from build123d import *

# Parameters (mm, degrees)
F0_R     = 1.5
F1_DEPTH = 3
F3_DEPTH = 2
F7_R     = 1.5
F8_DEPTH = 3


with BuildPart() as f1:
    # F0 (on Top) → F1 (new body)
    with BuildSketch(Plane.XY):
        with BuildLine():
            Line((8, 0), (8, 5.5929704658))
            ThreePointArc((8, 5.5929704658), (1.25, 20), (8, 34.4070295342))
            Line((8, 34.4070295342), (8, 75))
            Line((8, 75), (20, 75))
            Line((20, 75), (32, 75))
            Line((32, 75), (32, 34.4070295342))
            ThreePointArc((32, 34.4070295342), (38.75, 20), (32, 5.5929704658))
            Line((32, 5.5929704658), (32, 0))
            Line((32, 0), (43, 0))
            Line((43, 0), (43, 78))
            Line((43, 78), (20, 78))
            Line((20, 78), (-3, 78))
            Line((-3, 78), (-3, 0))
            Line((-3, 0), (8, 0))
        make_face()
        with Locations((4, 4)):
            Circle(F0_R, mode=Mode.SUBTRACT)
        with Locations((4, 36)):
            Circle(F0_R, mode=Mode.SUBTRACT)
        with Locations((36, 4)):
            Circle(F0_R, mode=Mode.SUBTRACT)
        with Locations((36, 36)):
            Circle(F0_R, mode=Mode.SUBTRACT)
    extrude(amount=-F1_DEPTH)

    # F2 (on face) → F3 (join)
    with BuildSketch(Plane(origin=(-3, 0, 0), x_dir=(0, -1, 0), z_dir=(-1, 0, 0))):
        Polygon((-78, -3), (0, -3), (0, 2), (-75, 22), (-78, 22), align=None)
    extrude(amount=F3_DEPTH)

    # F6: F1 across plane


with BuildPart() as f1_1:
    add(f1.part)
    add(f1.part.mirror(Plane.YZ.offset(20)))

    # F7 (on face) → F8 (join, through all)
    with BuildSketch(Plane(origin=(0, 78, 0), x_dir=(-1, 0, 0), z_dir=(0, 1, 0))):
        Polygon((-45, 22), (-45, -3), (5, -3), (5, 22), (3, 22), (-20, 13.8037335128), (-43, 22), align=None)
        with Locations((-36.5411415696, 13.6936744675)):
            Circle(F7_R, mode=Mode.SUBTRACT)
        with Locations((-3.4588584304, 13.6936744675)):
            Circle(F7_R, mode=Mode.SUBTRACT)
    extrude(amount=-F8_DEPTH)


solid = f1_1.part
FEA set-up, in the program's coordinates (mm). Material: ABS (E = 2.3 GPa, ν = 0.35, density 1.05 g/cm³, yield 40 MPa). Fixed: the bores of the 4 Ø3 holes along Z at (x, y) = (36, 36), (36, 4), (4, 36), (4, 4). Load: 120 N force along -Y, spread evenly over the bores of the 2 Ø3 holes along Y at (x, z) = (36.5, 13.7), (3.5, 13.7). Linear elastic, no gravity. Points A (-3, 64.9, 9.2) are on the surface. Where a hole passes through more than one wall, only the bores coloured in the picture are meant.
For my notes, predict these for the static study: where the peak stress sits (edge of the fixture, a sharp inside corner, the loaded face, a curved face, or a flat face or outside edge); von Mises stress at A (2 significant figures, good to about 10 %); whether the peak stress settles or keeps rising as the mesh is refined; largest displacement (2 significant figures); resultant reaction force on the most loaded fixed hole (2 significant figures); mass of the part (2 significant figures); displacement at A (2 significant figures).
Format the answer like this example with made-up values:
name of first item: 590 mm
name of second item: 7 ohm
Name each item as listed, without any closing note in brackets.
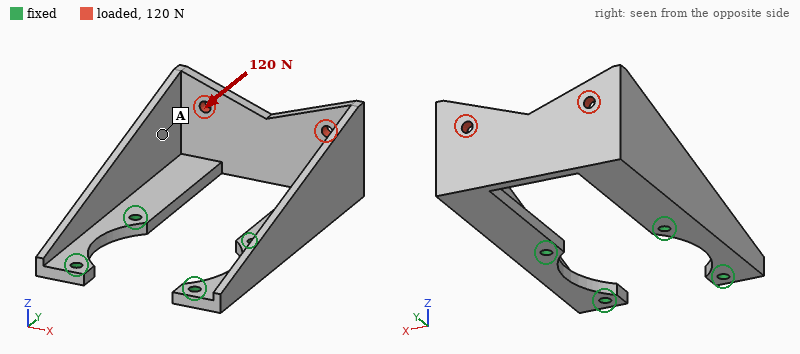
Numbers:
where the peak stress sits: a sharp inside corner
von Mises stress at A: 3.6 MPa
whether the peak stress settles or keeps rising as the mesh is refined: keeps rising
largest displacement: 0.91 mm
resultant reaction force on the most loaded fixed hole: 50 N
mass of the part: 12 g
displacement at A: 0.42 mm
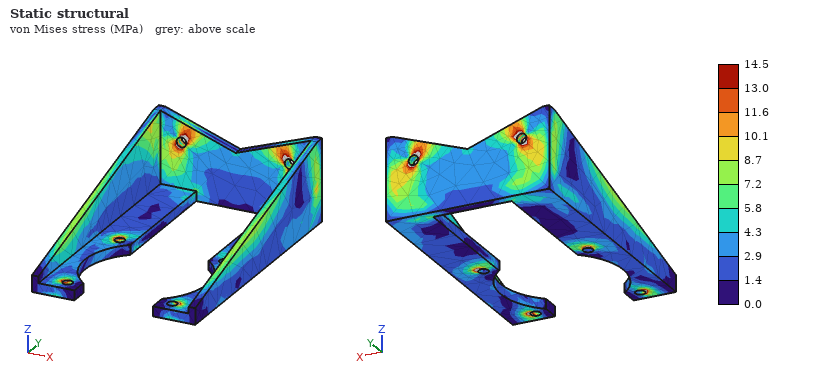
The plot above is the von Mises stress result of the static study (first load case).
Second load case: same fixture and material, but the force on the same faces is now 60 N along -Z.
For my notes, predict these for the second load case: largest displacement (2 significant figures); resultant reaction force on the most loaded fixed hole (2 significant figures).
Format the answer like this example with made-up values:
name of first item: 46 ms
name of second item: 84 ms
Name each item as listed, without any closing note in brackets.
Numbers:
largest displacement: 1.0 mm
resultant reaction force on the most loaded fixed hole: 74 N
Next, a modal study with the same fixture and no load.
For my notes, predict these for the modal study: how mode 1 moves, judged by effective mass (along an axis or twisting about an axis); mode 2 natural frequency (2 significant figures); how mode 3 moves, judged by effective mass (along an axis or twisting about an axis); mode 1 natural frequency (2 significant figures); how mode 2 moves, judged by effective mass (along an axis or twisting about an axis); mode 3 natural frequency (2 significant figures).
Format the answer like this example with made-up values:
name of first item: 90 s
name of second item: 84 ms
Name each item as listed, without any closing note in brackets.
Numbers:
how mode 1 moves, judged by effective mass: along X
mode 2 natural frequency: 550 Hz
how mode 3 moves, judged by effective mass: along X
mode 1 natural frequency: 520 Hz
how mode 2 moves, judged by effective mass: along Z
mode 3 natural frequency: 1000 Hz
